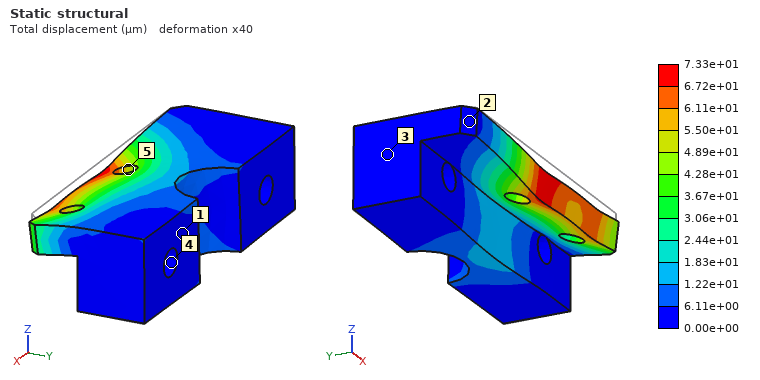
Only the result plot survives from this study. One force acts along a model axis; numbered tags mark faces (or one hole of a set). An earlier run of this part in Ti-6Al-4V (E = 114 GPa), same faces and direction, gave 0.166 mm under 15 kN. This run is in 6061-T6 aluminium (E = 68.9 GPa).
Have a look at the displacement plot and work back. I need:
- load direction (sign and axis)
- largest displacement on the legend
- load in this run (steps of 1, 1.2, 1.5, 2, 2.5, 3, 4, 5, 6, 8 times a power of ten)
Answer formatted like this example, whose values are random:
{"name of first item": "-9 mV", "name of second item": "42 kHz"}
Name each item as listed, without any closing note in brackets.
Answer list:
{"load direction": "-Z", "largest displacement on the legend": "7.33e+01 µm", "load in this run": "4 kN"}
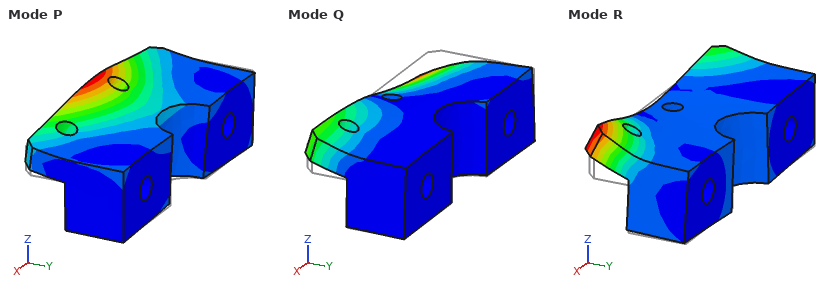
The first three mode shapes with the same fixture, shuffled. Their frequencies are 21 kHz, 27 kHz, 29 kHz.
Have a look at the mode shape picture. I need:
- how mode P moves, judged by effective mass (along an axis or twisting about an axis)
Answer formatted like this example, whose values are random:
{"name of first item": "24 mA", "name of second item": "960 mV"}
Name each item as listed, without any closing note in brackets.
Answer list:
{"how mode P moves, judged by effective mass": "along Z"}
